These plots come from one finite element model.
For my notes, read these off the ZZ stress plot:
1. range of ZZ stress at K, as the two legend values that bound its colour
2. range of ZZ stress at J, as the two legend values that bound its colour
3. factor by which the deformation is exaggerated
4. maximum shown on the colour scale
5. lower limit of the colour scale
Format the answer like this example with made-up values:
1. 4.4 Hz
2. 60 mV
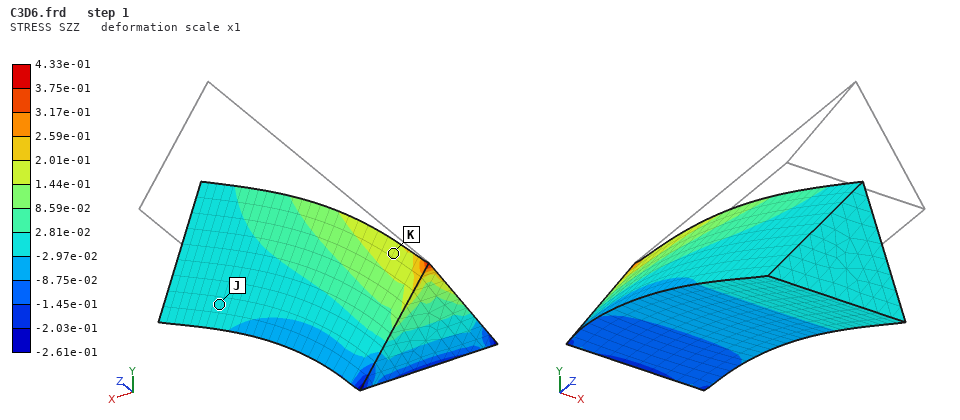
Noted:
1. 1.44e-01 to 2.01e-01
2. -2.97e-02 to 2.81e-02
3. 1
4. 4.33e-01
5. -2.61e-01
